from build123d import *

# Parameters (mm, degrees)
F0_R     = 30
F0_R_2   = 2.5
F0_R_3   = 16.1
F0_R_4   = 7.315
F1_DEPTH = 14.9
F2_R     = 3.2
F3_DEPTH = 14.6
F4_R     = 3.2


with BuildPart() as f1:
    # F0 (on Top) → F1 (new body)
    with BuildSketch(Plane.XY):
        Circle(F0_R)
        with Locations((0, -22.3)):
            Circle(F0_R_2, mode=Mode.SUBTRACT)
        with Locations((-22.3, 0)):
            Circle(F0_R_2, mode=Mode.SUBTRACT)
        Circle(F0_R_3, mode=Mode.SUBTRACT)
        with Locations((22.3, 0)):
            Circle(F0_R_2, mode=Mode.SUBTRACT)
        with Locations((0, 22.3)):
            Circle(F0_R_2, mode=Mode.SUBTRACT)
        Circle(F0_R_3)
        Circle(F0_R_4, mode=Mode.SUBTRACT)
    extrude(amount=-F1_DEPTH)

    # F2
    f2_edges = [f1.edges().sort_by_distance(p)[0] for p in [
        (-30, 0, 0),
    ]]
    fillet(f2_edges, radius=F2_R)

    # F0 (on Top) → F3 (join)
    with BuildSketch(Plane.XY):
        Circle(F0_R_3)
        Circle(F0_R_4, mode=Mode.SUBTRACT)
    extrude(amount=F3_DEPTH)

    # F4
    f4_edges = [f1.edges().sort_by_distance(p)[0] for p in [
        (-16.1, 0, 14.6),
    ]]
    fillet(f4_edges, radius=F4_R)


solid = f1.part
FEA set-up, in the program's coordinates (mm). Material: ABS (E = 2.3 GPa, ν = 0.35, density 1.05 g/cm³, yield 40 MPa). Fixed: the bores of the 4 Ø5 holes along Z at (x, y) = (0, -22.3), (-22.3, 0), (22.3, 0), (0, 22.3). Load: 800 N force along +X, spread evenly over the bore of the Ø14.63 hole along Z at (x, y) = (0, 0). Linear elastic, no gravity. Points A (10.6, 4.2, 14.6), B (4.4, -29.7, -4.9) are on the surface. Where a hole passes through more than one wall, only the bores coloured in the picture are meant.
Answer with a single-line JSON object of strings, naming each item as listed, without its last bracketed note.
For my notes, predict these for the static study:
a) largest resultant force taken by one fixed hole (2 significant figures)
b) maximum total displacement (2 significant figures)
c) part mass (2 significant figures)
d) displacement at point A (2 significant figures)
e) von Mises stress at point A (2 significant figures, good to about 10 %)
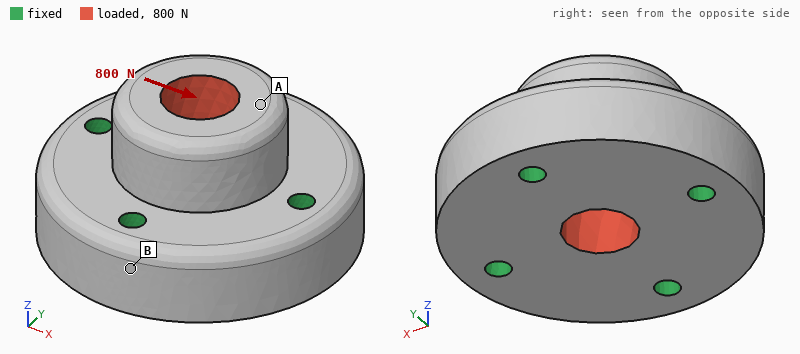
{"largest resultant force taken by one fixed hole": "280 N", "maximum total displacement": "25 µm", "part mass": "50 g", "displacement at point A": "23 µm", "von Mises stress at point A": "0.91 MPa"}
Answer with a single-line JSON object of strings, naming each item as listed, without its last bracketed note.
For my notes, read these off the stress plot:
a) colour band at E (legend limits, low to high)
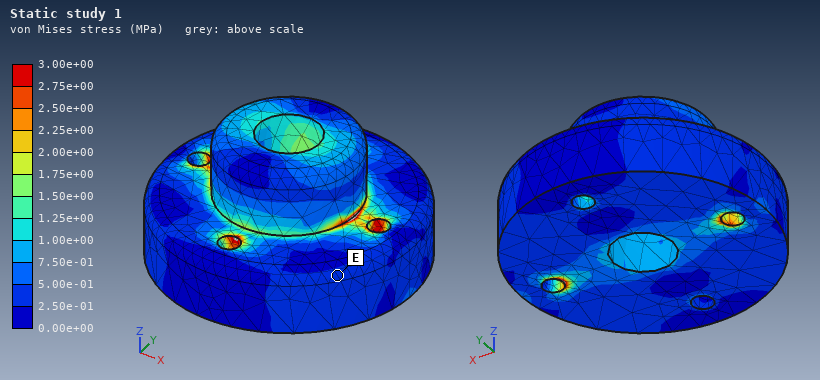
{"colour band at E": "2.50e-01 to 5.00e-01 MPa"}
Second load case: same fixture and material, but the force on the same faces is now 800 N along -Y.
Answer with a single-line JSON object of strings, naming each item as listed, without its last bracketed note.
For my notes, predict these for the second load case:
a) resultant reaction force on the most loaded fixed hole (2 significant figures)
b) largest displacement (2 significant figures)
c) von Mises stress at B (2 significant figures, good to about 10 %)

{"resultant reaction force on the most loaded fixed hole": "280 N", "largest displacement": "24 µm", "von Mises stress at B": "0.29 MPa"}
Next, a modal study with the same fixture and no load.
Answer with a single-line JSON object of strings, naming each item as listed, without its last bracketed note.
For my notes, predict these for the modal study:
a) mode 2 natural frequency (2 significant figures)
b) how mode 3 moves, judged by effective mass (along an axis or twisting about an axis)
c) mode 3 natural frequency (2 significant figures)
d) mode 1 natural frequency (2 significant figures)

{"mode 2 natural frequency": "7500 Hz", "how mode 3 moves, judged by effective mass": "along Z", "mode 3 natural frequency": "8400 Hz", "mode 1 natural frequency": "7500 Hz"}
